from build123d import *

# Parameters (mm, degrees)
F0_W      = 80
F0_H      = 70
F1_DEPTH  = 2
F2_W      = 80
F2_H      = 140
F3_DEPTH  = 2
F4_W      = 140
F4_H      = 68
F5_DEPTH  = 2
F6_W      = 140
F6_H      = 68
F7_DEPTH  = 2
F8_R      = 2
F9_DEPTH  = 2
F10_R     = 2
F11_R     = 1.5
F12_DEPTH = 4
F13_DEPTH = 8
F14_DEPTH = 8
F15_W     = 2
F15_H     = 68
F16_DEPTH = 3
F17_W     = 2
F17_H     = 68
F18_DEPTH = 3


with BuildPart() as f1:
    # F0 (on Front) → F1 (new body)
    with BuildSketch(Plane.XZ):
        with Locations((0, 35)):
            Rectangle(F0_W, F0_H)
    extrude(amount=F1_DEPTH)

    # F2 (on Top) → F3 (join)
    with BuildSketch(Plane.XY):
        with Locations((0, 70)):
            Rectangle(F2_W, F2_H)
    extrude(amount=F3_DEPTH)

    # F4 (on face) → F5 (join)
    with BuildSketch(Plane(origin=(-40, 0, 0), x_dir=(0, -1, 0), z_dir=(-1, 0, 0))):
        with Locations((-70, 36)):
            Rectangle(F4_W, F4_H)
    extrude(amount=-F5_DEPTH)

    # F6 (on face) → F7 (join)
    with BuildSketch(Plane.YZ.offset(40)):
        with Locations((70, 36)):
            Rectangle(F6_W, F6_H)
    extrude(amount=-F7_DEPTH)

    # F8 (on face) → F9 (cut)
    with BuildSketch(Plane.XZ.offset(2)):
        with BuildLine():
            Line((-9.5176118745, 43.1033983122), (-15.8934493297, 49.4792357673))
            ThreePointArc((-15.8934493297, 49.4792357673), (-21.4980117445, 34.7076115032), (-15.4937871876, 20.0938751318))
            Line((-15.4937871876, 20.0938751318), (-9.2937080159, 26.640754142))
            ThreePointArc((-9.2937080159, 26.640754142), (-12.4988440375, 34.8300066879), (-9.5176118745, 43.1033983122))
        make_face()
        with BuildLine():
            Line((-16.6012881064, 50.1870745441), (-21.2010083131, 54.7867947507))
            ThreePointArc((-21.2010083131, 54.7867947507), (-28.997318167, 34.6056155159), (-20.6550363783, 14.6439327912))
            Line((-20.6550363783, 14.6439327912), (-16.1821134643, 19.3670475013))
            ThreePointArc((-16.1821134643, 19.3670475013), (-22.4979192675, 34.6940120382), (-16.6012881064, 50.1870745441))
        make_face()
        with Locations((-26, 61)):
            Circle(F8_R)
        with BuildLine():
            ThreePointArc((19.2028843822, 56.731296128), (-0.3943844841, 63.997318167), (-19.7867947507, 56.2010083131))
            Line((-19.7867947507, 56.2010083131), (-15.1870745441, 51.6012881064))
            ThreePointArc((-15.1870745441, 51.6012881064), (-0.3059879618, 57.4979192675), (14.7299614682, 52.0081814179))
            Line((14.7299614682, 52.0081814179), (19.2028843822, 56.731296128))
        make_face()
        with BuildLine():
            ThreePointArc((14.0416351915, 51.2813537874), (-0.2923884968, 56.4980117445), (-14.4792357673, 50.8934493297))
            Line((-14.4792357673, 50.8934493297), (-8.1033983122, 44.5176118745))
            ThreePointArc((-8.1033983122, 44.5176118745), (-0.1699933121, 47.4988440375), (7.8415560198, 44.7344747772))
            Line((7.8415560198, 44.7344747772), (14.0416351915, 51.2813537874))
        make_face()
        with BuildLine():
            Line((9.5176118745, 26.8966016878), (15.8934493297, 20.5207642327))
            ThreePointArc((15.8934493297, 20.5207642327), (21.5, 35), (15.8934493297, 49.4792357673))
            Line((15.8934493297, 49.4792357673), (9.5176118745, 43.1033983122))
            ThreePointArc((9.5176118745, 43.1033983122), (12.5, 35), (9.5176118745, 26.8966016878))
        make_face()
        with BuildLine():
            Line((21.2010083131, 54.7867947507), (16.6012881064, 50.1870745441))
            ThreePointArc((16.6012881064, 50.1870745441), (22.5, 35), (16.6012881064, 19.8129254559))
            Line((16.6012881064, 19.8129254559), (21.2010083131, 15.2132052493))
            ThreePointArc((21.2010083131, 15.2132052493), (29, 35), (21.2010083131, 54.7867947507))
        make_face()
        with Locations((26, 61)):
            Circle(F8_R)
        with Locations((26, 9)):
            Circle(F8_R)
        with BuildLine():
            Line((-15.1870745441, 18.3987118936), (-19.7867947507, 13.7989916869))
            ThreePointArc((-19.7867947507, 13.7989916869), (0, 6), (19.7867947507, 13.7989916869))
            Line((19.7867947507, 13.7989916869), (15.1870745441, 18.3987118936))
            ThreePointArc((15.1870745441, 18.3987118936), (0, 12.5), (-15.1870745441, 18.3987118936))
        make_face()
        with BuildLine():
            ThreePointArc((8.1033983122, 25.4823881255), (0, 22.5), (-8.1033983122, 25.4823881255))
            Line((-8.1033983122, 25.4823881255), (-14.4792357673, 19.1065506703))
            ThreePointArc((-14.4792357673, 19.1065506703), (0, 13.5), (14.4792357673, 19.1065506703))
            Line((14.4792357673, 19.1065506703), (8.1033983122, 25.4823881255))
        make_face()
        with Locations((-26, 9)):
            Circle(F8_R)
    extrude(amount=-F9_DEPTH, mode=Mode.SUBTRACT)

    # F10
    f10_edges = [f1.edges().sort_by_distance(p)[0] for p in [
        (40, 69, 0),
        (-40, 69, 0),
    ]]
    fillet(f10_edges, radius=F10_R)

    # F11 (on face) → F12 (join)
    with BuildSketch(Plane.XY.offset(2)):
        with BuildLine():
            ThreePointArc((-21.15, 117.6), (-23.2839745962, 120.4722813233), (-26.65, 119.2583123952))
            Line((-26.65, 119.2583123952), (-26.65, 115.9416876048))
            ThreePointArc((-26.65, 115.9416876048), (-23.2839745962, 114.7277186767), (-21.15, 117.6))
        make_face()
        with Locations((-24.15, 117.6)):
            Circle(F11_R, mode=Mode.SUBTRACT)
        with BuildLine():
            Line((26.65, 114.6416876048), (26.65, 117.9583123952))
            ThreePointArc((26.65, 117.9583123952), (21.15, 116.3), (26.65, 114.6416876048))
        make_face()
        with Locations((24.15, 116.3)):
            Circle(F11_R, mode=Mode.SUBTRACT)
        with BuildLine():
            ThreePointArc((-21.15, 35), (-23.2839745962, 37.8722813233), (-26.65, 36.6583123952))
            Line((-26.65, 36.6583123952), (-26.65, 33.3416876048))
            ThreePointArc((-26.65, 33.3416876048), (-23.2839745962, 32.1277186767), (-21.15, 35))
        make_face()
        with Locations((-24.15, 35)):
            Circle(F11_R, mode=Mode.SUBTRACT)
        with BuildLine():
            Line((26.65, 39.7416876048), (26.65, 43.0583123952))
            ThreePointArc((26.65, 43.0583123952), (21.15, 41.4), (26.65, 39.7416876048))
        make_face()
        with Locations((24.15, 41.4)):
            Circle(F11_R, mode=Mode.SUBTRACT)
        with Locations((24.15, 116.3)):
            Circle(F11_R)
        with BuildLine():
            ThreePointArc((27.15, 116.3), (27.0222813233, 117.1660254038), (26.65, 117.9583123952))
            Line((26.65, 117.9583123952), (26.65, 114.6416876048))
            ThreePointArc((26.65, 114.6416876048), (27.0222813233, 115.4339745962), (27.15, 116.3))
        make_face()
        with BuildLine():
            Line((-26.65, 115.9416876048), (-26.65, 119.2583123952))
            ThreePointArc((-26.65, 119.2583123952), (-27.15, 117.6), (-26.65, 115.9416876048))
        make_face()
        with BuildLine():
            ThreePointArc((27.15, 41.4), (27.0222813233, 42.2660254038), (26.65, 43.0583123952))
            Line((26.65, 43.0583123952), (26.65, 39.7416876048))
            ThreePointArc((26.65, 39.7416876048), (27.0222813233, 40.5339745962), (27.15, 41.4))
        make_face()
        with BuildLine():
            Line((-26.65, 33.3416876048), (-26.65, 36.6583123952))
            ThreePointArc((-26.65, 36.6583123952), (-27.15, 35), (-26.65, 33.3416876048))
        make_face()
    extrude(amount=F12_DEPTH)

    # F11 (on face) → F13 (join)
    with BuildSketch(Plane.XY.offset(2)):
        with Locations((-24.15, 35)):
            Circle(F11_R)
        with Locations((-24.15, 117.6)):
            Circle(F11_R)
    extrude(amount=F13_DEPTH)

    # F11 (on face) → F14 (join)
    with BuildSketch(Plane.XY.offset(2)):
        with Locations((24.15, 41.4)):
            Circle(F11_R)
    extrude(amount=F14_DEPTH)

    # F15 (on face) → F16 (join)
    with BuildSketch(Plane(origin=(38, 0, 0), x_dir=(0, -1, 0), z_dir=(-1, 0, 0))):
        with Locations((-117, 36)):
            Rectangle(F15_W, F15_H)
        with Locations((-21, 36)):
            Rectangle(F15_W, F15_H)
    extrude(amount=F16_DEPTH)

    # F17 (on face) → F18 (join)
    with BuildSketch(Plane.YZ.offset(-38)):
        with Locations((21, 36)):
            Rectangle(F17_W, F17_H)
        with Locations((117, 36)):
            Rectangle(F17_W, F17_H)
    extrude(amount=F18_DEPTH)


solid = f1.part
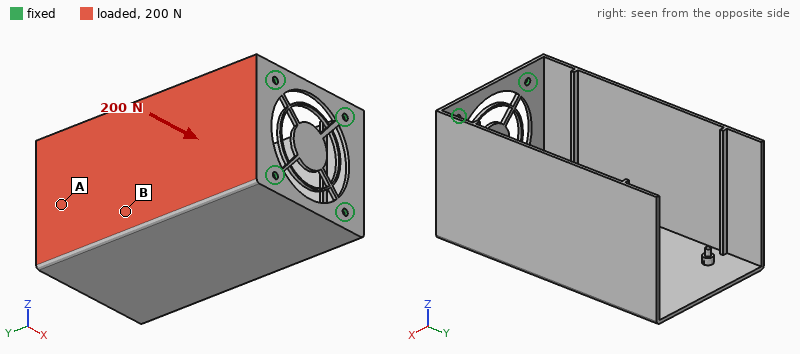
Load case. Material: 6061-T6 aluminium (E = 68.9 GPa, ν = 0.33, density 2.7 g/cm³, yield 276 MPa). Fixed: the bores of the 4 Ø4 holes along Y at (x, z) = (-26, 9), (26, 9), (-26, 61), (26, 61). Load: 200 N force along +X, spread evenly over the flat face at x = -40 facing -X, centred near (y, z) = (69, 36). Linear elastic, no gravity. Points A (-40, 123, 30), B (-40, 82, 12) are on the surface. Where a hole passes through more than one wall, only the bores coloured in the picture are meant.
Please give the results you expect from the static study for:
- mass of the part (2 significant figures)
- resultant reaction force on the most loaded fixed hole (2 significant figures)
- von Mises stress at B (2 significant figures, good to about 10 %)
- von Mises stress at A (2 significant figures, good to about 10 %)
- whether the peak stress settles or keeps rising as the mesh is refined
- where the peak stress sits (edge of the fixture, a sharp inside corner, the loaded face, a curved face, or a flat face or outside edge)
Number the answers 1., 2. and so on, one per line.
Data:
1. 190 g
2. 350 N
3. 23 MPa
4. 11 MPa
5. keeps rising
6. edge of the fixture
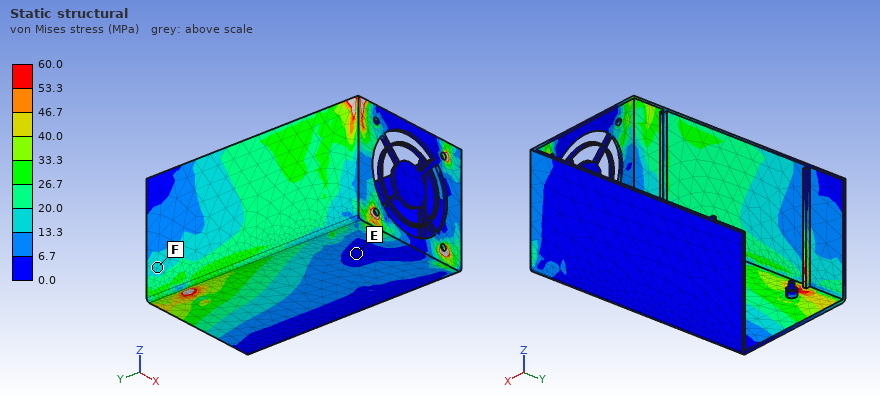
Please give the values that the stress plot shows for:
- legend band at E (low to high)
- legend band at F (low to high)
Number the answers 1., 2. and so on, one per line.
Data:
1. 0.0 to 6.7 MPa
2. 13.3 to 20.0 MPa
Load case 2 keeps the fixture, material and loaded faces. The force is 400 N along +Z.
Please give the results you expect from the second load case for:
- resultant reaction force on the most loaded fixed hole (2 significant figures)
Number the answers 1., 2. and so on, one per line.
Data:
1. 550 N
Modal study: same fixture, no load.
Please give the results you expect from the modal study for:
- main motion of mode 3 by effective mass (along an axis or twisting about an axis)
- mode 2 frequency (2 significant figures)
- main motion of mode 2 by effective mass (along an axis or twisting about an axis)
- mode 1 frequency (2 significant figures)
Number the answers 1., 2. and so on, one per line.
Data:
1. along Z
2. 310 Hz
3. along X
4. 280 Hz
